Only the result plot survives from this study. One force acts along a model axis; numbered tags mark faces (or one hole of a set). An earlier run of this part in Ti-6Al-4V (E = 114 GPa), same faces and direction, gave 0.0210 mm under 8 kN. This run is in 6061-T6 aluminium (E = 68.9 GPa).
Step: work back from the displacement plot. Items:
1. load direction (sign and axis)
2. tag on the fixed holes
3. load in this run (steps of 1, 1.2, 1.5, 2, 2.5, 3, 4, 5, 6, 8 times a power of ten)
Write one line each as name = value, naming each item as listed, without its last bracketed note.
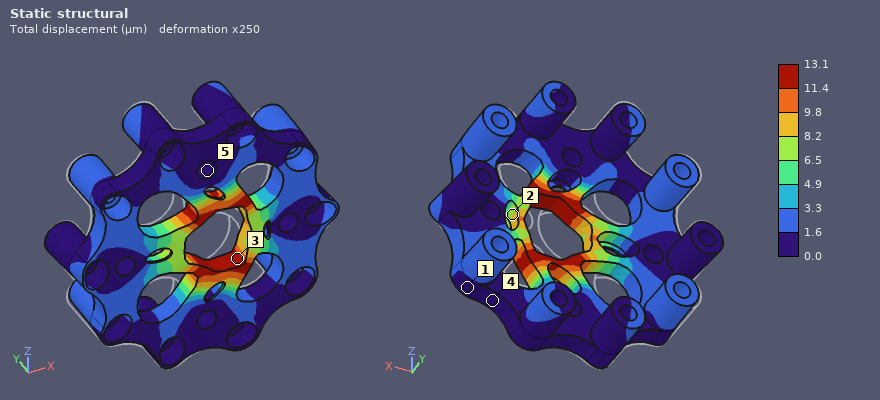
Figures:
load direction = +X
tag on the fixed holes = 5
load in this run = 3 kN
